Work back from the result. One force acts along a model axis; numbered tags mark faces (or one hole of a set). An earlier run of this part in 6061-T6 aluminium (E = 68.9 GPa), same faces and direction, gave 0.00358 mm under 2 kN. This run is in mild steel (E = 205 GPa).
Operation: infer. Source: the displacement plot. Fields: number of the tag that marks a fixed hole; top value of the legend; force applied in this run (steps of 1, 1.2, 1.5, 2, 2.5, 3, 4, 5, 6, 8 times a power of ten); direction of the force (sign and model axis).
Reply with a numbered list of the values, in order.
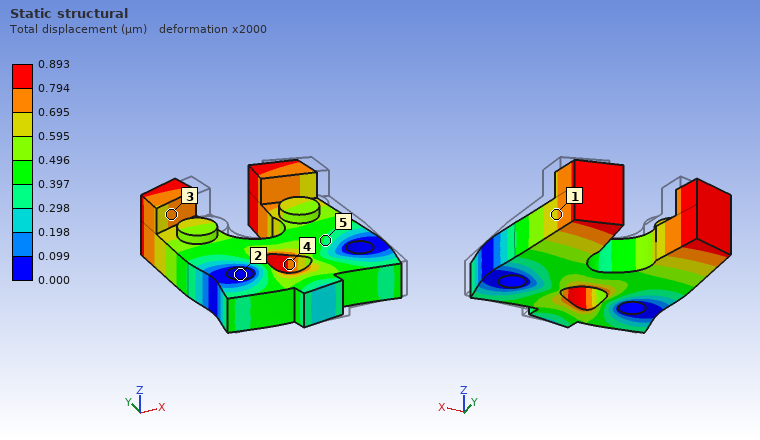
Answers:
1. 2
2. 0.893 µm
3. 1.5 kN
4. -X
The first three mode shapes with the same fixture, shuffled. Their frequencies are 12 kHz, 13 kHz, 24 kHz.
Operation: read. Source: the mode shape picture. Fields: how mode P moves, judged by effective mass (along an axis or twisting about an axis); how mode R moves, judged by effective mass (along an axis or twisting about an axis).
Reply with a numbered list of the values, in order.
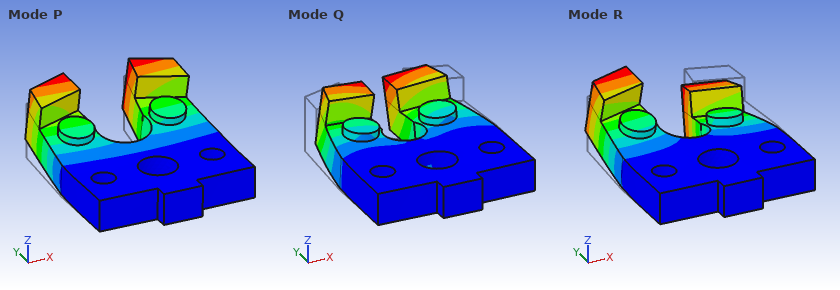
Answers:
1. along Z
2. twisting about Y
